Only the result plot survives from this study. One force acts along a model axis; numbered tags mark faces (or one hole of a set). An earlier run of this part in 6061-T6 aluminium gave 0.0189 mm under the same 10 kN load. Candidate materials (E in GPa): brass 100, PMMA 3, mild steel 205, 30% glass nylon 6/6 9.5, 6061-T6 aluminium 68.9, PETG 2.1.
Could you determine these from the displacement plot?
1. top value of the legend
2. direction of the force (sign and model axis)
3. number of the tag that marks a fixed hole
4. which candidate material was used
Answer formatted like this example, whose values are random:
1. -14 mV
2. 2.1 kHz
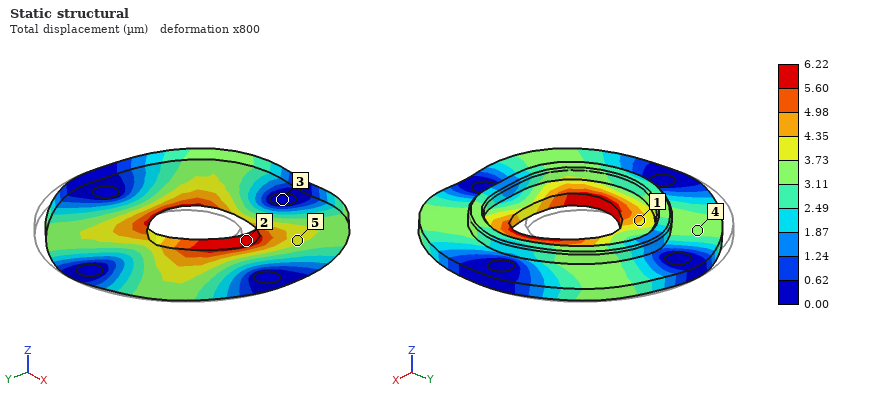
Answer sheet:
1. 6.22 µm
2. -Y
3. 3
4. mild steel
